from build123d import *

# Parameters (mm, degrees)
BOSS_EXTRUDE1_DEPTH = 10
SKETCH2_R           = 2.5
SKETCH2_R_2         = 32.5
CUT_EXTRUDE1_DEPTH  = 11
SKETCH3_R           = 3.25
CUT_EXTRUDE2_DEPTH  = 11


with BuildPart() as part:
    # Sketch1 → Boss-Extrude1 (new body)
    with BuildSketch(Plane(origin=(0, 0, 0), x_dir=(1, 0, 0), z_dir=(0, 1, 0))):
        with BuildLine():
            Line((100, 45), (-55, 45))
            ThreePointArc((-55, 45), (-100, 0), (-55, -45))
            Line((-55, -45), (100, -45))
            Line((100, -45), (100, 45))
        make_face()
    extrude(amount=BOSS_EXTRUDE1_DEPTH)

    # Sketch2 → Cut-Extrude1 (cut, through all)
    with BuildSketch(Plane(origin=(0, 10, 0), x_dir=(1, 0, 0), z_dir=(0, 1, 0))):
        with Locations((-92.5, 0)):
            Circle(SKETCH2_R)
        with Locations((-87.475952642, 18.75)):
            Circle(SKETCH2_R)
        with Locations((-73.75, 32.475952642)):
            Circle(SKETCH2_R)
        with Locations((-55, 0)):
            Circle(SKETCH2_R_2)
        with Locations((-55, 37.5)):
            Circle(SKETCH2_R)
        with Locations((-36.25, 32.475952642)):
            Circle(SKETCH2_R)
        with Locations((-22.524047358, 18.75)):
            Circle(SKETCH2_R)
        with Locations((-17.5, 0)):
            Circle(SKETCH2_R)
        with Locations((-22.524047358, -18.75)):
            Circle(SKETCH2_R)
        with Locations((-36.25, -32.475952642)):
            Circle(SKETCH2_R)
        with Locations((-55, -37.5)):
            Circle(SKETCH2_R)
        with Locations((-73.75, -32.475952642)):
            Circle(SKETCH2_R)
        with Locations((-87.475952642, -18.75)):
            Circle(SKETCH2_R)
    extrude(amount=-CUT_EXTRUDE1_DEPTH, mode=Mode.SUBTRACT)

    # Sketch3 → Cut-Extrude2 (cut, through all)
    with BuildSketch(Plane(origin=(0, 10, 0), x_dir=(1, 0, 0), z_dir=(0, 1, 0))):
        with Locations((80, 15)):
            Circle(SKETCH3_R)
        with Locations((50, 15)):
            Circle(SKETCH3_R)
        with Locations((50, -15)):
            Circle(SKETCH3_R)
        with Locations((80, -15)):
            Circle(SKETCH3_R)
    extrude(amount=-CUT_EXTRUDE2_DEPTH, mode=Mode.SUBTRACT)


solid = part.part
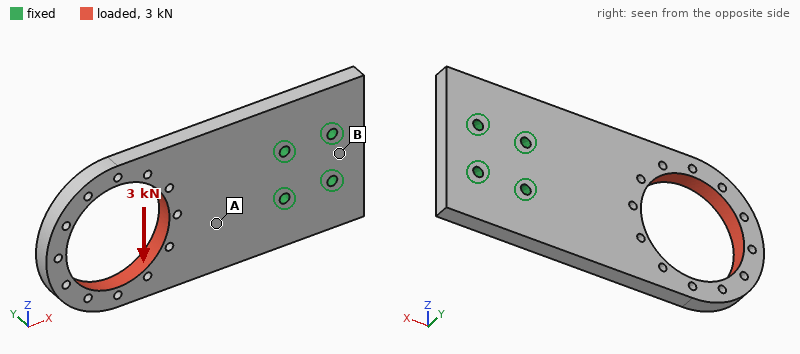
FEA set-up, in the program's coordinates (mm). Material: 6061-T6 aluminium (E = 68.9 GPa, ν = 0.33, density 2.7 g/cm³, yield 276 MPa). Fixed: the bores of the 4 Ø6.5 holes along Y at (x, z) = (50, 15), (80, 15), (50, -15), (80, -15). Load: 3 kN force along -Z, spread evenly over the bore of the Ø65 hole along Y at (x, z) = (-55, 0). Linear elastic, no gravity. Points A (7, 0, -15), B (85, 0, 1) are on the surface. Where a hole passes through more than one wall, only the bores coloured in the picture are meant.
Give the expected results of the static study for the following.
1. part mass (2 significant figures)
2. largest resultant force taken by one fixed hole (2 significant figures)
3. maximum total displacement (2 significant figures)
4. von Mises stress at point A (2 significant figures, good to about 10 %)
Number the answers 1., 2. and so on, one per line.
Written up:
1. 360 g
2. 5.3 kN
3. 0.20 mm
4. 9.2 MPa
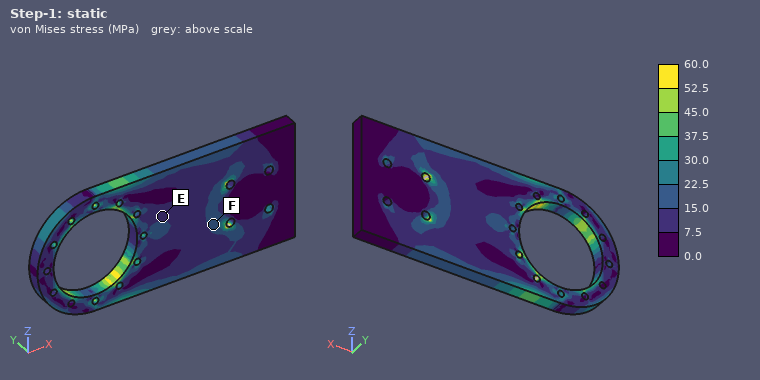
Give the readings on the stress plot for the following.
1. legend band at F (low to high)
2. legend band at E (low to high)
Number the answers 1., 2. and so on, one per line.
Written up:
1. 15.0 to 22.5 MPa
2. 7.5 to 15.0 MPa
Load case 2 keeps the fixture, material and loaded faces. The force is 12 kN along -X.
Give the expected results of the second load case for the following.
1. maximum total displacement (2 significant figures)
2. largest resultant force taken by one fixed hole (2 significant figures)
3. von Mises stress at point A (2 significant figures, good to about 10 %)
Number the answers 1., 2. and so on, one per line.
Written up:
1. 0.11 mm
2. 4.6 kN
3. 11 MPa
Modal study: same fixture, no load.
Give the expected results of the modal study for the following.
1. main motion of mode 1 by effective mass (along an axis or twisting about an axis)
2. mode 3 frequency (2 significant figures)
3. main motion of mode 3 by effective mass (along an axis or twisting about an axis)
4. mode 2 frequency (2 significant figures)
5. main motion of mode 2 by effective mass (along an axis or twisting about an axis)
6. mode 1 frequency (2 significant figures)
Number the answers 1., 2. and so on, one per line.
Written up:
1. along Y
2. 1900 Hz
3. along Y
4. 1400 Hz
5. twisting about X
6. 530 Hz
